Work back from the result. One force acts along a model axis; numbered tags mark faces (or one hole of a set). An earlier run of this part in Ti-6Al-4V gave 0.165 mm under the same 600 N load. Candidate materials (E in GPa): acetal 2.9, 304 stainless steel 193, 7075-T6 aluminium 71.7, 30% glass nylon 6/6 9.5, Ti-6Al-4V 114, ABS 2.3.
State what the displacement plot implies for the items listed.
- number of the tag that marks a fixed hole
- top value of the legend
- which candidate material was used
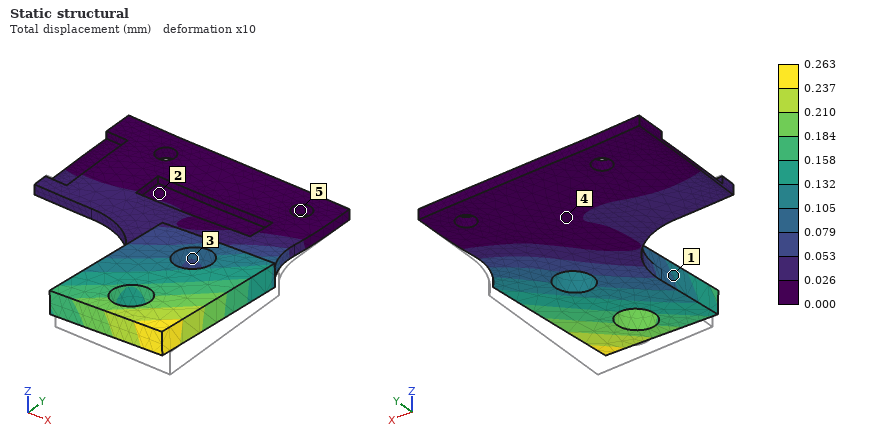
5
0.263 mm
7075-T6 aluminium
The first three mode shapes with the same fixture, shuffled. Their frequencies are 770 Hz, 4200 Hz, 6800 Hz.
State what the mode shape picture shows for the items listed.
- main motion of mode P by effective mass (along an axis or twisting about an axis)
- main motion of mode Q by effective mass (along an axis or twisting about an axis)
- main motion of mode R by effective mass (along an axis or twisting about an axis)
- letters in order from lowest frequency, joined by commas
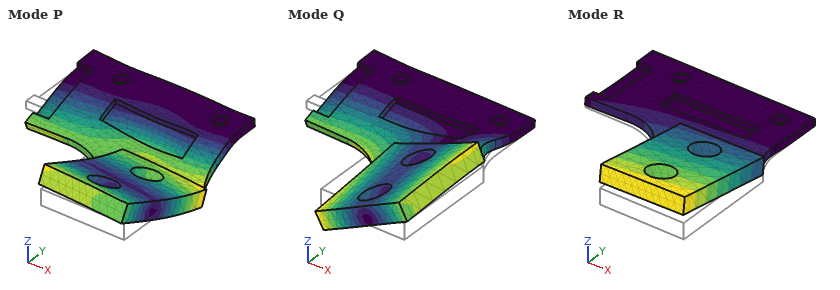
along Z
twisting about Y
along Z
R, Q, P
